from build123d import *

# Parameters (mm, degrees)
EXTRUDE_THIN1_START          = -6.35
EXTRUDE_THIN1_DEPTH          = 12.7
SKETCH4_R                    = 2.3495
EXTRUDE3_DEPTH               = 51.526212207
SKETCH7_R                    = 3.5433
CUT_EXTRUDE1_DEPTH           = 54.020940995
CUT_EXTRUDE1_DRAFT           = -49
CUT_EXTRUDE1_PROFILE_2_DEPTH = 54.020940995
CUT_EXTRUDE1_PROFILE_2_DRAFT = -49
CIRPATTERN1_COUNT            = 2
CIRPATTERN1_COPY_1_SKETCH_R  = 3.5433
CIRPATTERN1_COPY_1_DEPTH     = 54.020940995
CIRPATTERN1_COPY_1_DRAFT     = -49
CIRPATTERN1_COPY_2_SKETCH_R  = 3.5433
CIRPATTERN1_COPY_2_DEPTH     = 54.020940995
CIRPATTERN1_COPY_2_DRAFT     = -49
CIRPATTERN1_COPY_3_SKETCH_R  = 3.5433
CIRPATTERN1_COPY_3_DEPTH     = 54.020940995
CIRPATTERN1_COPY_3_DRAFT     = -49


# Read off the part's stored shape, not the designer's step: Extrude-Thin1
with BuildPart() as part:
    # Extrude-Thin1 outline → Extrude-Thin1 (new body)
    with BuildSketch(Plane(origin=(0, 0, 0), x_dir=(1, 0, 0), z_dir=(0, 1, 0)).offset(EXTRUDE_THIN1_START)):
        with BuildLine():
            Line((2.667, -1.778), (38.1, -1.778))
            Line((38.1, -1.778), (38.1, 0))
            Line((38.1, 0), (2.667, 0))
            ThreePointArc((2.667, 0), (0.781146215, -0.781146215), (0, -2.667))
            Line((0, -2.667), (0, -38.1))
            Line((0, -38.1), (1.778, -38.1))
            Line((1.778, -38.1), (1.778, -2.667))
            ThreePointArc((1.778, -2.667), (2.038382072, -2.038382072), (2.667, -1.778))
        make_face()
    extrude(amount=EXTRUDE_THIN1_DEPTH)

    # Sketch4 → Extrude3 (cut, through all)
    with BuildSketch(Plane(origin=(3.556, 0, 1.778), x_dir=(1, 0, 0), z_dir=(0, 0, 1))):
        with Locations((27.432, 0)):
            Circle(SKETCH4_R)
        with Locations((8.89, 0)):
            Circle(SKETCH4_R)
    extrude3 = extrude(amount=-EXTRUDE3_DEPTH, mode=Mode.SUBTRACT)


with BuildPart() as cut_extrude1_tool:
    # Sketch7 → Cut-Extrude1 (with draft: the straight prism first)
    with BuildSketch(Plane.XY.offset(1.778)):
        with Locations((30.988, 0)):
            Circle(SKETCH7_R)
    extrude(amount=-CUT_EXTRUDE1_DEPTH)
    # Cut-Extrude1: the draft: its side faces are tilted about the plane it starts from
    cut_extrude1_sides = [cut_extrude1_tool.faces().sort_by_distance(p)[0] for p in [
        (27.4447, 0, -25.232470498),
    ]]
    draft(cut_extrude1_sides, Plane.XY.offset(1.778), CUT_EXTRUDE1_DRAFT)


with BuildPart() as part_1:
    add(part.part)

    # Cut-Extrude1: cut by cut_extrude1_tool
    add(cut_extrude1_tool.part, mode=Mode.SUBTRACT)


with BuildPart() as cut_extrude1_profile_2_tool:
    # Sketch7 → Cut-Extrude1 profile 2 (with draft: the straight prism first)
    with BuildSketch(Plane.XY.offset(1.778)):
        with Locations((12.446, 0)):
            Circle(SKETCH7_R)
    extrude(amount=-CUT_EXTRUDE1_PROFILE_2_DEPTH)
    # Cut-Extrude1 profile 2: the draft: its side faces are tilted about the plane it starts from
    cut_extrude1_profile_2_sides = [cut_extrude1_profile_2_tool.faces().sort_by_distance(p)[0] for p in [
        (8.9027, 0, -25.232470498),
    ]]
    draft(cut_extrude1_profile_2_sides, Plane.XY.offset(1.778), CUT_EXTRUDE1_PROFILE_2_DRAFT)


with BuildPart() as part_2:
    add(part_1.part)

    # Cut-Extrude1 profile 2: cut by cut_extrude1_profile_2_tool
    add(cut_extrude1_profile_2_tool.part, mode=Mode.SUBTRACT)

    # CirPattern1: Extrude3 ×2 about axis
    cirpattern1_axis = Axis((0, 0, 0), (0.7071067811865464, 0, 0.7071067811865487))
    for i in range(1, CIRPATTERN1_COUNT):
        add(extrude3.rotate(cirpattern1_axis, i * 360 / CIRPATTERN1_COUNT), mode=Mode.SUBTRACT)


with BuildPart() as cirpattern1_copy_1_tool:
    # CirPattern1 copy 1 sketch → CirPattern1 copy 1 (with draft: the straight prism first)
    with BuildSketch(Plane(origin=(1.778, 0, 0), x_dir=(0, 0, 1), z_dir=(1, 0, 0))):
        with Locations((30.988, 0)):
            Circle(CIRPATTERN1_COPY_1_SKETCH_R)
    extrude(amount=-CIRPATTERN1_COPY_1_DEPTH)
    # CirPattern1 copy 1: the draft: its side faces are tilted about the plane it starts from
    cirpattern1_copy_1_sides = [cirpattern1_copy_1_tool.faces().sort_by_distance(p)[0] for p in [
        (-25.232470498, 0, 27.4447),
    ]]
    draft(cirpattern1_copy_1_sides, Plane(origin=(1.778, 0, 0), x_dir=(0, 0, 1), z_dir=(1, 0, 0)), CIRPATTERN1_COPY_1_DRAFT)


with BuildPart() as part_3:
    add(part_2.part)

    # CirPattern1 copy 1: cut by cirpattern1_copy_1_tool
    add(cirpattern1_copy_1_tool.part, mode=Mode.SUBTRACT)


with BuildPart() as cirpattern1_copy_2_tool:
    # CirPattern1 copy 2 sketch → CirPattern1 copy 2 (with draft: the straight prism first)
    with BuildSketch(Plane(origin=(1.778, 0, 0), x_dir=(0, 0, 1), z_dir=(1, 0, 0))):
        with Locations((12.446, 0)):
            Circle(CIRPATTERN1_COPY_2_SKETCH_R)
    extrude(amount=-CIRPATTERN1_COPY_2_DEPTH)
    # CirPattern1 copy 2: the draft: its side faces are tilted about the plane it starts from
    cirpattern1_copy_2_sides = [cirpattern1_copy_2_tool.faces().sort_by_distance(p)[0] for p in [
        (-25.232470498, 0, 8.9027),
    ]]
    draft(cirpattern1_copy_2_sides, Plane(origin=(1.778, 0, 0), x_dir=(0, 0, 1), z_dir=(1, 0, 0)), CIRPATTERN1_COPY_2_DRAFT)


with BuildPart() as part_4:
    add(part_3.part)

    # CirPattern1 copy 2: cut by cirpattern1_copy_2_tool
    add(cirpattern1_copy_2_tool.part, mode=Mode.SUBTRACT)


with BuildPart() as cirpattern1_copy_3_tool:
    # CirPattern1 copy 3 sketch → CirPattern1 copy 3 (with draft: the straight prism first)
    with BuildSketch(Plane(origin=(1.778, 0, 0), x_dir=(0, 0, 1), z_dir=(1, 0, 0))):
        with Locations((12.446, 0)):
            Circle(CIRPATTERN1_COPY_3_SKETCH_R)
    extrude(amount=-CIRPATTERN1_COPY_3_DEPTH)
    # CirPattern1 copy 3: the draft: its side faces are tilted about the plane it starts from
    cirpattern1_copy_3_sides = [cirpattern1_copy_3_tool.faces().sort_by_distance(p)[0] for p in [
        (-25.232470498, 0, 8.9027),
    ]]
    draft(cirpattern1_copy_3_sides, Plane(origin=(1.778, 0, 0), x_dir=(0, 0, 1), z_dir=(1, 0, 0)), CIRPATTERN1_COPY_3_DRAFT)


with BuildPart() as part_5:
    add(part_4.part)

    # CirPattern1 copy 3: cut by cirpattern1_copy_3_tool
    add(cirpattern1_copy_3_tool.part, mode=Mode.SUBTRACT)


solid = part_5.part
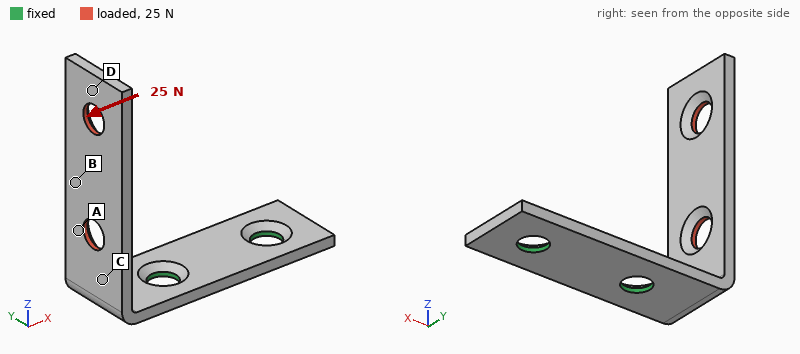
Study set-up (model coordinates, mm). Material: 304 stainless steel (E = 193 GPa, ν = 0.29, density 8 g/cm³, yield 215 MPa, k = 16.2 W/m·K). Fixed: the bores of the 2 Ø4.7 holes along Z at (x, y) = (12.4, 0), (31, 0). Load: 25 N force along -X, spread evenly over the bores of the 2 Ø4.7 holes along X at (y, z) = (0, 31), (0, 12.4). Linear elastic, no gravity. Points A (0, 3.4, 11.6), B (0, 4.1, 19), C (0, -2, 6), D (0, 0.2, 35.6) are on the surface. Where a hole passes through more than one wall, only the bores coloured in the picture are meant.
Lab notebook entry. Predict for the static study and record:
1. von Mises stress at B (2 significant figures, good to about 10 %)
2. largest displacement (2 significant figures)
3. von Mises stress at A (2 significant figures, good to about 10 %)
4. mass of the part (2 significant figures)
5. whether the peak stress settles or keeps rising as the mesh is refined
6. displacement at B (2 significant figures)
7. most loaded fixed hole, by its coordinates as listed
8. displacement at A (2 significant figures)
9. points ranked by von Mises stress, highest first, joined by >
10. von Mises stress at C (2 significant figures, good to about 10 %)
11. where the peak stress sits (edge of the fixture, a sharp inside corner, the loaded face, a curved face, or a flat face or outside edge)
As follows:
23 MPa
0.37 mm
65 MPa
12 g
keeps rising
0.16 mm
(31, 0)
0.086 mm
A > C > B > D
52 MPa
edge of the fixture
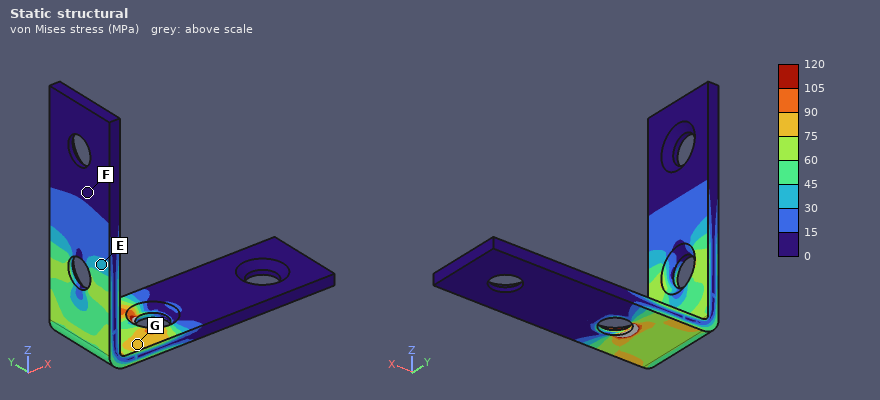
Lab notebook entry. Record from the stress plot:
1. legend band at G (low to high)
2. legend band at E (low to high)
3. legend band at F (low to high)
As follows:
75 to 90 MPa
30 to 45 MPa
0 to 15 MPa
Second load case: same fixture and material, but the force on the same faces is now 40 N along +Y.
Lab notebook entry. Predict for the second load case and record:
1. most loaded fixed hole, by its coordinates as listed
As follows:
(12.4, 0)
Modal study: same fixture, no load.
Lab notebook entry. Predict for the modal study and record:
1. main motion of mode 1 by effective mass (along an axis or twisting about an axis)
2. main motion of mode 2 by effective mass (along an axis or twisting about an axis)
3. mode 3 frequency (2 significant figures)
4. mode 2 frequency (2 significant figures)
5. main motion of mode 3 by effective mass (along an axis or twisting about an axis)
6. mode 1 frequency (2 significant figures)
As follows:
along X
along Y
3400 Hz
1200 Hz
along Z
690 Hz
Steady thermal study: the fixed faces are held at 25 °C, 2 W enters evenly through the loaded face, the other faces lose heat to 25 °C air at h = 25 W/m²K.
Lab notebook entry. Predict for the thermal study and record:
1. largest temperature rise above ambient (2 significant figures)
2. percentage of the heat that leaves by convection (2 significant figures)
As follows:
70 K
69 %
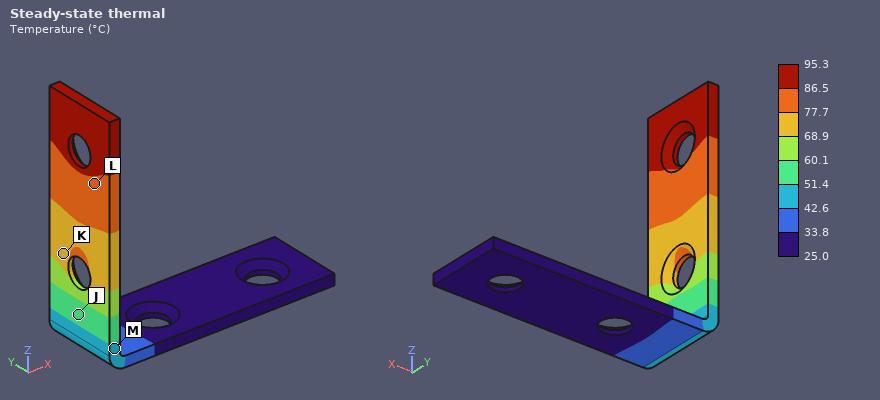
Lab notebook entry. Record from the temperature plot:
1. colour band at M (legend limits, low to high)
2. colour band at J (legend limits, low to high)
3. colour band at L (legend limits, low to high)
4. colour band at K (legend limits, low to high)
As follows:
42.6 to 51.4 °C
51.4 to 60.1 °C
77.7 to 86.5 °C
68.9 to 77.7 °C
